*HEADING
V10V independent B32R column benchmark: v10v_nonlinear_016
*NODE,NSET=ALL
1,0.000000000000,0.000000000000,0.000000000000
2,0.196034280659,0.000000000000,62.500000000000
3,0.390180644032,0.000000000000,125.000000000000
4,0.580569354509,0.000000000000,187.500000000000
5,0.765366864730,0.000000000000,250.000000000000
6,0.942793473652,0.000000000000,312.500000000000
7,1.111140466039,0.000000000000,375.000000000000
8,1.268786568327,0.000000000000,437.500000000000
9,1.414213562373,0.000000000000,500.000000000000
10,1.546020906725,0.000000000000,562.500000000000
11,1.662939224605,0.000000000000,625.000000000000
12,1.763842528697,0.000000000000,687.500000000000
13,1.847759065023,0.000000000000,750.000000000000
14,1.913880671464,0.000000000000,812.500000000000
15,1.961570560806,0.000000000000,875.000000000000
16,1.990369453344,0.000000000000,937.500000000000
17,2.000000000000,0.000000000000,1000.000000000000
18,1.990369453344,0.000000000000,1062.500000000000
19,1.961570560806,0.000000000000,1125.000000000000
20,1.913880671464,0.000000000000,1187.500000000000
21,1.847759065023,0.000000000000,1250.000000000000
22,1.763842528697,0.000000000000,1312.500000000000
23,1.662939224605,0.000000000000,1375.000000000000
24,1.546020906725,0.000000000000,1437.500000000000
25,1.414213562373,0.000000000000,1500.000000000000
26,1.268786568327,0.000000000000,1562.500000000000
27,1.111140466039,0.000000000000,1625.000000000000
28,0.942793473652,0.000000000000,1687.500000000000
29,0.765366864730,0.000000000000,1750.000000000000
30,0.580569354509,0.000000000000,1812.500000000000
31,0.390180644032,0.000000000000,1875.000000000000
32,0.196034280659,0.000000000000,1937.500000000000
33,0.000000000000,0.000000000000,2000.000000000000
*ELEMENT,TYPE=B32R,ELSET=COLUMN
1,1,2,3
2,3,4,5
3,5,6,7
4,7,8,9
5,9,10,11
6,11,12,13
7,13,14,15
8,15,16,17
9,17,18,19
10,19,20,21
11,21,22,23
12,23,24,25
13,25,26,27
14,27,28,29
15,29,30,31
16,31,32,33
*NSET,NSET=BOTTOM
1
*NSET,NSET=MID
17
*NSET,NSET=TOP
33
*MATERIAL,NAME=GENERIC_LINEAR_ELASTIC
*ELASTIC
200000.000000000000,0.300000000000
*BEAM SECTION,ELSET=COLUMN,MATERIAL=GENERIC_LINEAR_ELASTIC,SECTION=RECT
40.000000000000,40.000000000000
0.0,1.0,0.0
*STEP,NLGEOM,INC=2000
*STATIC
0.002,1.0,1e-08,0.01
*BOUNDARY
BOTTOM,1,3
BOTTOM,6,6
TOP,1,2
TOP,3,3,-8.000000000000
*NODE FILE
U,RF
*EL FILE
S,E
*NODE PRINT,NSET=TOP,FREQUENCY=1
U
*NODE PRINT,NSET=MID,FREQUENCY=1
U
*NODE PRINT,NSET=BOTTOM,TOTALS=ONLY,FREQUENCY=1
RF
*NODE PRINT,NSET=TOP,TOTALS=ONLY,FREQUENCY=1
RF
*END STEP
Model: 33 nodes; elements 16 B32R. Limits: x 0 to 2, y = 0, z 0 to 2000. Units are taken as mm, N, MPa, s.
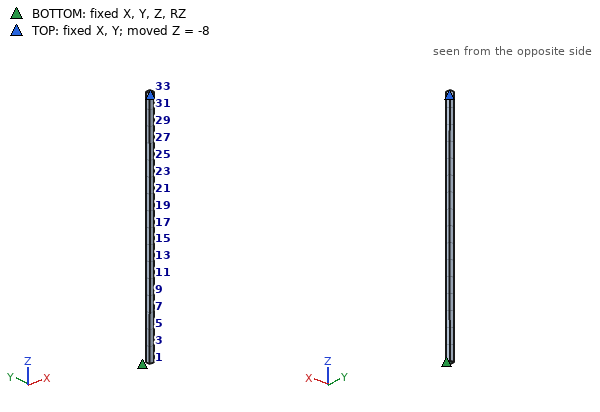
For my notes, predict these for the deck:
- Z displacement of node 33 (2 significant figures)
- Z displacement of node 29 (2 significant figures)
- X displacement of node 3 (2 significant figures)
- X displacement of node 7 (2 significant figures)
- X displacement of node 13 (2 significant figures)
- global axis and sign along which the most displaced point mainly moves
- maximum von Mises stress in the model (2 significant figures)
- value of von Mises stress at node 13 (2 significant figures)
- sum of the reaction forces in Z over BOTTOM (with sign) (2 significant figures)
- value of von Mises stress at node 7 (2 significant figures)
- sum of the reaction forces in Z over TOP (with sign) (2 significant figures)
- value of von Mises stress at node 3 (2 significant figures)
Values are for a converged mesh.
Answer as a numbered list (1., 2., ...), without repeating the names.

1. -10 mm
2. -8.3 mm
3. 15 mm
4. 42 mm
5. 69 mm
6. +X
7. 800 MPa
8. 750 MPa
9. 1.0e+05 N
10. 480 MPa
11. -1.0e+05 N
12. 210 MPa
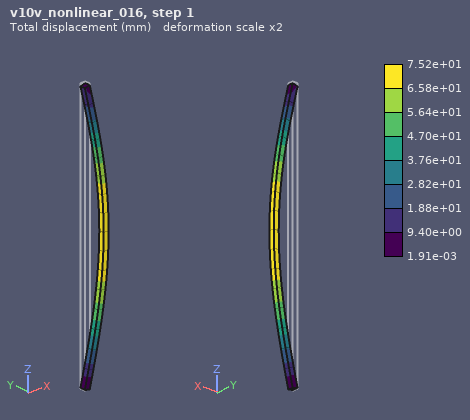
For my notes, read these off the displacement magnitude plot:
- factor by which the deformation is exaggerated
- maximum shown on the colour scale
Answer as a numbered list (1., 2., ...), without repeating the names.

1. 2
2. 7.52e+01 mm
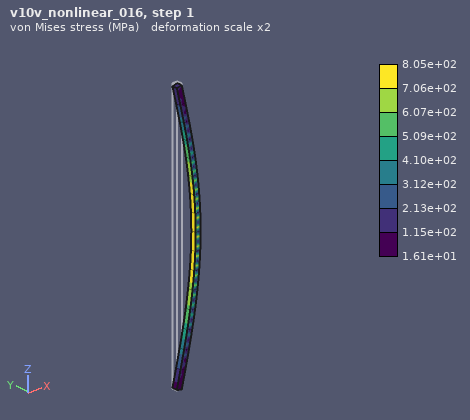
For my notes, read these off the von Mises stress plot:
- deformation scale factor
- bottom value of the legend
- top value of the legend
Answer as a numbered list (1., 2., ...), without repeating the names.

1. 2
2. 1.61e+01 MPa
3. 8.05e+02 MPa
